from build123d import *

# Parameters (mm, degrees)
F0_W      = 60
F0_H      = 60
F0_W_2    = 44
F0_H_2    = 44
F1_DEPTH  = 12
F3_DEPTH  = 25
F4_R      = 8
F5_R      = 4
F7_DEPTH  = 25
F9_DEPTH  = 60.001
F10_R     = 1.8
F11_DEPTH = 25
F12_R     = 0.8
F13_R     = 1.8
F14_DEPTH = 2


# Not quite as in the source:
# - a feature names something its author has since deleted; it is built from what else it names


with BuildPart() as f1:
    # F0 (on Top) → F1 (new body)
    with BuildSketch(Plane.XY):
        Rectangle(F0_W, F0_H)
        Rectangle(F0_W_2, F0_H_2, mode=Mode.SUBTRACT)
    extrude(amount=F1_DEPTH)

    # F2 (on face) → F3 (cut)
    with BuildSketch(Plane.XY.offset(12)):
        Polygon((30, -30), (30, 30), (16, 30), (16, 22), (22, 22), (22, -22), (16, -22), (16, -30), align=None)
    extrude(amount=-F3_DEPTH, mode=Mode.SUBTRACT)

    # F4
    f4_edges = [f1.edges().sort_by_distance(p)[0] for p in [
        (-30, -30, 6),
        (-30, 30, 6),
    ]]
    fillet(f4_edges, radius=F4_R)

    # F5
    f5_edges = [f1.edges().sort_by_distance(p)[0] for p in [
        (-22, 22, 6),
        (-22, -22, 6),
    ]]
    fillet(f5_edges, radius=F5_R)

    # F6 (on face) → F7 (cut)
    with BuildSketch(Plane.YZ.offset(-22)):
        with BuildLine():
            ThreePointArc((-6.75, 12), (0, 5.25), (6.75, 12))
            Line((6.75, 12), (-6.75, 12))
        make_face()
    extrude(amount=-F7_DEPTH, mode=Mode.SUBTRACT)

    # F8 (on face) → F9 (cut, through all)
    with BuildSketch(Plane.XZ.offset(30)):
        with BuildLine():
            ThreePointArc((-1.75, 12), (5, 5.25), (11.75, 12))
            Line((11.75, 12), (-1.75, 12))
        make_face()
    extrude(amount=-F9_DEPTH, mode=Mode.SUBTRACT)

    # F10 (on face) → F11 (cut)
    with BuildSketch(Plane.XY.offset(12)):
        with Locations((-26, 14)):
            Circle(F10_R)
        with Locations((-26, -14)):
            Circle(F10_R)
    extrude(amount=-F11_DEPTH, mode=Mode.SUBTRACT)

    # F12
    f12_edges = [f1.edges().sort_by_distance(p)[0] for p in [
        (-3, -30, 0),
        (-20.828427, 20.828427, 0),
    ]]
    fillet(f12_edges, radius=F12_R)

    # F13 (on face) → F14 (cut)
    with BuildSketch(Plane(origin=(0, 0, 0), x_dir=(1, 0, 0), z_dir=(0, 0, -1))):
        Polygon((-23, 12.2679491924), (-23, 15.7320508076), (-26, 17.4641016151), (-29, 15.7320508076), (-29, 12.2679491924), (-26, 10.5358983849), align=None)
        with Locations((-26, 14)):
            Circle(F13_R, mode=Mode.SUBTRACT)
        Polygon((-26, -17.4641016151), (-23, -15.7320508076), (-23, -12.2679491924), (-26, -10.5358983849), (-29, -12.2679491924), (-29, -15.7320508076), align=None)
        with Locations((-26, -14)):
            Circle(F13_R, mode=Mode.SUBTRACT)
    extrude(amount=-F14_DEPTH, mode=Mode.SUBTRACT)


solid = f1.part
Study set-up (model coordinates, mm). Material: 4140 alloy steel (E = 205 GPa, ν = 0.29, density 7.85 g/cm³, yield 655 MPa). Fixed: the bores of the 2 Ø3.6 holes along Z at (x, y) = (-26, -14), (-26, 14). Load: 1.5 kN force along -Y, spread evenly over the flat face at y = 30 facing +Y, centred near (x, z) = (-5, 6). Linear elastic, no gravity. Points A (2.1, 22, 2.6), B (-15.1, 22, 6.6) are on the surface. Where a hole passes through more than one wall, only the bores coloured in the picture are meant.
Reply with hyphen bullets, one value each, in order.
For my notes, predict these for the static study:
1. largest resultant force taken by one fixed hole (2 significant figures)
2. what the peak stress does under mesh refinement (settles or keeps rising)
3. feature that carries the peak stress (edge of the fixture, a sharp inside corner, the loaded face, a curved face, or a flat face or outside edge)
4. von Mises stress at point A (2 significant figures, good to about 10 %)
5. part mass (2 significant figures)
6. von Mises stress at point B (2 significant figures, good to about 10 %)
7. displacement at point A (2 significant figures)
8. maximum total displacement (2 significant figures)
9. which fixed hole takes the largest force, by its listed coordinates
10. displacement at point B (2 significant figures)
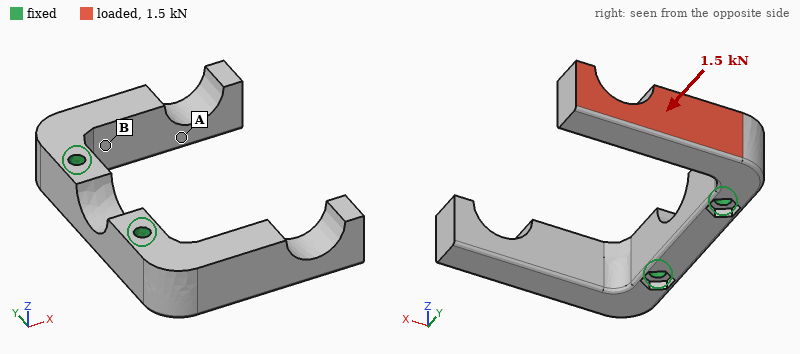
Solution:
- 1.5 kN
- keeps rising
- edge of the fixture
- 66 MPa
- 84 g
- 130 MPa
- 0.15 mm
- 0.25 mm
- (-26, 14)
- 0.043 mm
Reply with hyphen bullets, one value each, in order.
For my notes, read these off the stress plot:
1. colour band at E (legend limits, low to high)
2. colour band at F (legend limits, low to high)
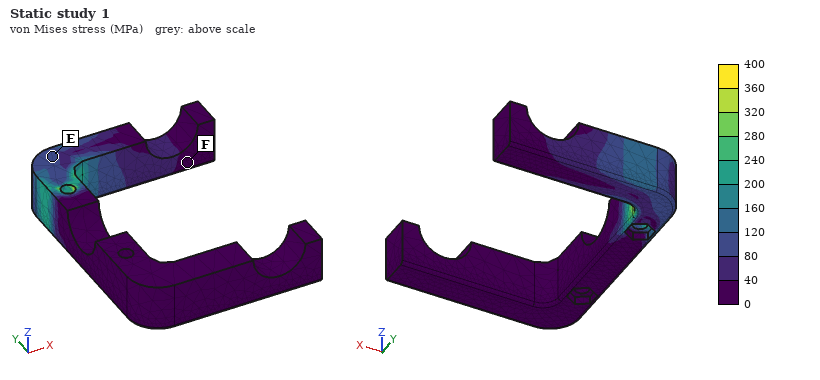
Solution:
- 80 to 120 MPa
- 0 to 40 MPa
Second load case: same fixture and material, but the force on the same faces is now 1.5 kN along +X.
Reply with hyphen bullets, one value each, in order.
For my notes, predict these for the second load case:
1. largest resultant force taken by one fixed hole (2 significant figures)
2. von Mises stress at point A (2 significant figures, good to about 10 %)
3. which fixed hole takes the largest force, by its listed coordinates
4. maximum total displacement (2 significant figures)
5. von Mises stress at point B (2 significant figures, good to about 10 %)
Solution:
- 1.7 kN
- 22 MPa
- (-26, 14)
- 0.12 mm
- 24 MPa
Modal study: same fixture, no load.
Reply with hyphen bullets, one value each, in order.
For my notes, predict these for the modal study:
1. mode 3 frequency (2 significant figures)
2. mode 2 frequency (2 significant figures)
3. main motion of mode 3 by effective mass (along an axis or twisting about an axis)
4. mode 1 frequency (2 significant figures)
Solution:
- 3600 Hz
- 3100 Hz
- along Z
- 3000 Hz
